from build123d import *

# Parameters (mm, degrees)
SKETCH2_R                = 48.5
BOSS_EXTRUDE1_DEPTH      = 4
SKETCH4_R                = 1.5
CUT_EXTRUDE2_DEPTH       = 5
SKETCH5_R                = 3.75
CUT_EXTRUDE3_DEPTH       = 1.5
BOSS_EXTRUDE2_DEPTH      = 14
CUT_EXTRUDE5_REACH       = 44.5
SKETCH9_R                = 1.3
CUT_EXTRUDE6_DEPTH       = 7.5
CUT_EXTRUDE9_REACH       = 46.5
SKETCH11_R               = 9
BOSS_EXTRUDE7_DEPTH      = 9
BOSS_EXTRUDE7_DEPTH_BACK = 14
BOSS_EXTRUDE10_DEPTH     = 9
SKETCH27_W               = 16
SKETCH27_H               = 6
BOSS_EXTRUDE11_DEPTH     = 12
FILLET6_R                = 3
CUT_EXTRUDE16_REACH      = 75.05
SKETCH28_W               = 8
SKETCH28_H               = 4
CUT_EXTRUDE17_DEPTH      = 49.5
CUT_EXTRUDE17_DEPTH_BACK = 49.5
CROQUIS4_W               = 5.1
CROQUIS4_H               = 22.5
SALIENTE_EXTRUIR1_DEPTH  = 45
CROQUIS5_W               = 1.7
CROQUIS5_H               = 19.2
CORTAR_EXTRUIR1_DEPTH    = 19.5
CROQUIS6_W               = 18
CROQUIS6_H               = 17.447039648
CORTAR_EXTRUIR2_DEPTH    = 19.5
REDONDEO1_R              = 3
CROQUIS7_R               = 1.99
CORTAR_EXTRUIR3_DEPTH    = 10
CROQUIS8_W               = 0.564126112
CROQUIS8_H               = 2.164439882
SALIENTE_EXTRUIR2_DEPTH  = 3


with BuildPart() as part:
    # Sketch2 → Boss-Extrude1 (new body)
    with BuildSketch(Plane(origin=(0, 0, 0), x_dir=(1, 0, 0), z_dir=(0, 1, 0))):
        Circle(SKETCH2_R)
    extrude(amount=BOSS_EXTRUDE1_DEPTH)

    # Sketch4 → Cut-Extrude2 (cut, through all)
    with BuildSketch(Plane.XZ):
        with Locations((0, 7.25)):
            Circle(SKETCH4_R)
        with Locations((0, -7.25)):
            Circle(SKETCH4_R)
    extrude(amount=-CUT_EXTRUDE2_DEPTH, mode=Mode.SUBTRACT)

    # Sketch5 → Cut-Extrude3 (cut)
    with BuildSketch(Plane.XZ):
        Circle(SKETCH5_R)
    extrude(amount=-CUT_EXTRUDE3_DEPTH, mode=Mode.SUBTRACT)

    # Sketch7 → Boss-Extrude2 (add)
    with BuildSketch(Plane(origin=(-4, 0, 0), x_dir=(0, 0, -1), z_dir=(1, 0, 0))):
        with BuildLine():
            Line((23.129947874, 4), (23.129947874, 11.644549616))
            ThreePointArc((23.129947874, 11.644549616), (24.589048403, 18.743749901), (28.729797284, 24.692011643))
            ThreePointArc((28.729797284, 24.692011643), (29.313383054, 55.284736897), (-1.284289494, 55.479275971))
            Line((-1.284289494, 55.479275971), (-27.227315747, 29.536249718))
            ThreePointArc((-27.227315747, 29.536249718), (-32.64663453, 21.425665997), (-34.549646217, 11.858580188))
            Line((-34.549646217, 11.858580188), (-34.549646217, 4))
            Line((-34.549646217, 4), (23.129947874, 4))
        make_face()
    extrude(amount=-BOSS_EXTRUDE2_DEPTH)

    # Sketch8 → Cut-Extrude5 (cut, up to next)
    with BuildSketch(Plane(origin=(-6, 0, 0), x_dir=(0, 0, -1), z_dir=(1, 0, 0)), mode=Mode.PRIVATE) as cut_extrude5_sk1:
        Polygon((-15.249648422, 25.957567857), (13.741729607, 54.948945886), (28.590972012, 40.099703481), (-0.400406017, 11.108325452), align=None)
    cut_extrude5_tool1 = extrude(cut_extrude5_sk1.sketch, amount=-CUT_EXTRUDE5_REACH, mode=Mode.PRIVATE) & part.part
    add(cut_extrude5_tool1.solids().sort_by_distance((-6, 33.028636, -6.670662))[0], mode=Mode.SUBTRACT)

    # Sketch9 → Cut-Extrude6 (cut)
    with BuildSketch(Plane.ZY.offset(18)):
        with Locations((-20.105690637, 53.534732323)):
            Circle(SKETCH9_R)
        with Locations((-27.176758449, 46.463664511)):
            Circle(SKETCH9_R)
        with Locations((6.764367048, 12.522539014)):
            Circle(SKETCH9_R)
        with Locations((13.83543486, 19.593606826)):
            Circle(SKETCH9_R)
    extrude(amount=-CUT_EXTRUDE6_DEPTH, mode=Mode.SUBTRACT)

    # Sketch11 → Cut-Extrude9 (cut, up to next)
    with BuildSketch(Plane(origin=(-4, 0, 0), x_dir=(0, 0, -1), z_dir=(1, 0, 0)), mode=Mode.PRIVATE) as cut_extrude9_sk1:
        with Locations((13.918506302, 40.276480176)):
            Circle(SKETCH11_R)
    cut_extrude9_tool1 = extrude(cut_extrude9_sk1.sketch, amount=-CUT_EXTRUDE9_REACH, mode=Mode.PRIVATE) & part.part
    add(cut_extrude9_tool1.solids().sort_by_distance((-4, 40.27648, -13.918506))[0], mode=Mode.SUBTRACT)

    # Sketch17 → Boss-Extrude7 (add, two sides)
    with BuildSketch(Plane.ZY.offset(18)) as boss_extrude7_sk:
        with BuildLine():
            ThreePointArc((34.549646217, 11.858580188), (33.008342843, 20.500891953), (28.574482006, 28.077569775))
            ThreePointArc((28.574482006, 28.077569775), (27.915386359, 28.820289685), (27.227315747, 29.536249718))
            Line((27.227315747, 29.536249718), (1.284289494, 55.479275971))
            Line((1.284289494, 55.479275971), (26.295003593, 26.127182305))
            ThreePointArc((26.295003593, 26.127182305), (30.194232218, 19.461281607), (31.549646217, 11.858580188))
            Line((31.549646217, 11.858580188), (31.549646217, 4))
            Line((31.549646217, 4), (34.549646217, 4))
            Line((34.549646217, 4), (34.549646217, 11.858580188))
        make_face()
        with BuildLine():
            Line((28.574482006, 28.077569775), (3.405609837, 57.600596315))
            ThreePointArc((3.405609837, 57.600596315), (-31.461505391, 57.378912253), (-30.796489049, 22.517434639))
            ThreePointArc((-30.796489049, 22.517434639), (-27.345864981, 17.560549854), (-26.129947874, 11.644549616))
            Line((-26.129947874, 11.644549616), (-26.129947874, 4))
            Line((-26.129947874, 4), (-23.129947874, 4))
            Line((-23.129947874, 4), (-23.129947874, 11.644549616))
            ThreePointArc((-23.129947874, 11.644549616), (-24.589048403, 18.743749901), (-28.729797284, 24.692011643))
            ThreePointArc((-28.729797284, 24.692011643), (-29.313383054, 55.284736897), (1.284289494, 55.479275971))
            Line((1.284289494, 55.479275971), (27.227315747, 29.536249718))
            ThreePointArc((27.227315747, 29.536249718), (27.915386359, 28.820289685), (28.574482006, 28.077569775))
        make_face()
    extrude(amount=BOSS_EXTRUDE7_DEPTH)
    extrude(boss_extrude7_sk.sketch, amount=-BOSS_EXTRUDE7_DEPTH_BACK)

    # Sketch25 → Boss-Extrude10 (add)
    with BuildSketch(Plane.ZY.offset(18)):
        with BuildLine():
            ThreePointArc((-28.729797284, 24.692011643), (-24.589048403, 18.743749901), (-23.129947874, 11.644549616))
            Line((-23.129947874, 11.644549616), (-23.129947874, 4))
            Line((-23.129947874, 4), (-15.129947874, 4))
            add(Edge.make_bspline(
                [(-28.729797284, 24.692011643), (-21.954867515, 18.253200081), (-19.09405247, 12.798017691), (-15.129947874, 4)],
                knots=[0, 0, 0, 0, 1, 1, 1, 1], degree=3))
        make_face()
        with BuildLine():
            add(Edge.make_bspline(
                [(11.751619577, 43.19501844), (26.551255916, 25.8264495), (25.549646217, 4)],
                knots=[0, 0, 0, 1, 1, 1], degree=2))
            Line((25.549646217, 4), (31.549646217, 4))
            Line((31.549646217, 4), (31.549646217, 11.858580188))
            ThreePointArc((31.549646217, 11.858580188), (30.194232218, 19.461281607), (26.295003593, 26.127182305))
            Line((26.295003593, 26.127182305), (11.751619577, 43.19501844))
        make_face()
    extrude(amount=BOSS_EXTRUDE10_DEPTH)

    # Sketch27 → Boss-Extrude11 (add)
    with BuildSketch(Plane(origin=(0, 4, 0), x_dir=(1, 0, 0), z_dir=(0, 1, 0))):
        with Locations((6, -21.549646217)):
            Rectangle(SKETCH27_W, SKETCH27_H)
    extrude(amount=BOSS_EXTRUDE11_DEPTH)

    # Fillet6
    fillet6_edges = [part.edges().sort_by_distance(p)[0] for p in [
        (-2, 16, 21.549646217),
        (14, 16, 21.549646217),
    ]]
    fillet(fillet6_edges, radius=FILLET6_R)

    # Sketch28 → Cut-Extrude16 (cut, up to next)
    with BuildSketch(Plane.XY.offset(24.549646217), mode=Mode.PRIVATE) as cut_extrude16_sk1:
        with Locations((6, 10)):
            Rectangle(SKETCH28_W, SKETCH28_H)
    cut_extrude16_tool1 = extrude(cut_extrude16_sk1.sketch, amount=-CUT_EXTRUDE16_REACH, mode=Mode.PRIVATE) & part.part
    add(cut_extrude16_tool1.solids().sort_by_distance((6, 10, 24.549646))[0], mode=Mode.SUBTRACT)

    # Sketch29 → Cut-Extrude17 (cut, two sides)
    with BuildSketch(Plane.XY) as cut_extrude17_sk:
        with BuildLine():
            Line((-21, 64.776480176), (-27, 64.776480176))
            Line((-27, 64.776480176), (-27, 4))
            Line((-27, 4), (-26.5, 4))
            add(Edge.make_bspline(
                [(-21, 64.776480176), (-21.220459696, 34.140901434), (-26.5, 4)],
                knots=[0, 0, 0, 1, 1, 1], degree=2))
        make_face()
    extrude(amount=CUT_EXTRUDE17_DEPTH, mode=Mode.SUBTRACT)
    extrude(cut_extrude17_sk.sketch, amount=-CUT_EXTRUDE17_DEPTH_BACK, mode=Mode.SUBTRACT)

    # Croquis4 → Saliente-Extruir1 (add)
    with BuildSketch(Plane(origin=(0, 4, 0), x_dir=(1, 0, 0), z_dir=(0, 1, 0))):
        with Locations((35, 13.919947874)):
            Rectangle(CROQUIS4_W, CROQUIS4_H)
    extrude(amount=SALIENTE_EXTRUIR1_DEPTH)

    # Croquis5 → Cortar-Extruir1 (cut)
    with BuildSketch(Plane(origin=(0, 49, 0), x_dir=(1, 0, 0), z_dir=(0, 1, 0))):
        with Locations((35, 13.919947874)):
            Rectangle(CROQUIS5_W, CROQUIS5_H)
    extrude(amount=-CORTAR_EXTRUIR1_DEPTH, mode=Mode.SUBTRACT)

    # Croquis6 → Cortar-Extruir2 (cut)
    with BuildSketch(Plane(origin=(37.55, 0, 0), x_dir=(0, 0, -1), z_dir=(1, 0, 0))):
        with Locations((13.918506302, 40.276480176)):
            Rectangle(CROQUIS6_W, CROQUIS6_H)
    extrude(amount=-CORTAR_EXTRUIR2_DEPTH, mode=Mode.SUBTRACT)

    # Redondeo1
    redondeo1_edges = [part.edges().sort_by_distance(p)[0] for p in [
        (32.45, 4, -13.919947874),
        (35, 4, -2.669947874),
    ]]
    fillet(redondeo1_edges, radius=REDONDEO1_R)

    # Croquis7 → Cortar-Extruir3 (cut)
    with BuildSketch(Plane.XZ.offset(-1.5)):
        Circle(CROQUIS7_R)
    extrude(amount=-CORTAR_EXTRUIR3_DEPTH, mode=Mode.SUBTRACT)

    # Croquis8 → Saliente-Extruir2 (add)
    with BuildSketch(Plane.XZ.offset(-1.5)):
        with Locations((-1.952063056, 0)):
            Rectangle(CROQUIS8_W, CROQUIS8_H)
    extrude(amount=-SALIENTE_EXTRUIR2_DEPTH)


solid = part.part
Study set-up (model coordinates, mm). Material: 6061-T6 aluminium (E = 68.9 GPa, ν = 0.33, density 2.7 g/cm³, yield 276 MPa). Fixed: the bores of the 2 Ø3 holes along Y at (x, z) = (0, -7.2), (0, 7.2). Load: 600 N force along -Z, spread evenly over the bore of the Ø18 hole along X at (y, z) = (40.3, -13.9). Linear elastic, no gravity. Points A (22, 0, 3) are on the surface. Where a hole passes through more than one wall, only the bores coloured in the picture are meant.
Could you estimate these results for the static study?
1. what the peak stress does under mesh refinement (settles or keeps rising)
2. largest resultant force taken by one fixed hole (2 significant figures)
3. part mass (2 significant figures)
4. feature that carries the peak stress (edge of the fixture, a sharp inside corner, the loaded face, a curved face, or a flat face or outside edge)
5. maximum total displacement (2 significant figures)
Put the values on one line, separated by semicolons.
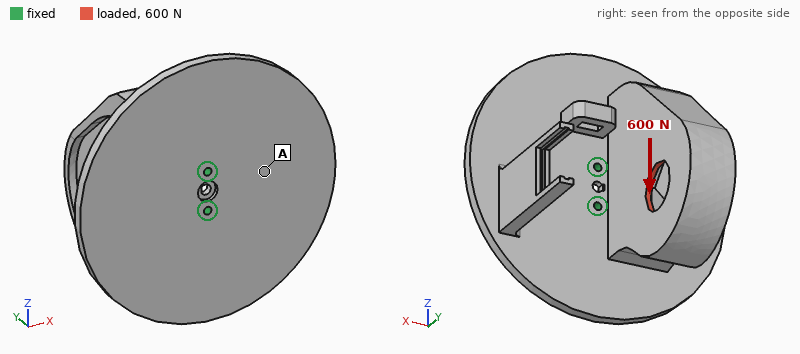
keeps rising; 1.3 kN; 190 g; edge of the fixture; 0.10 mm
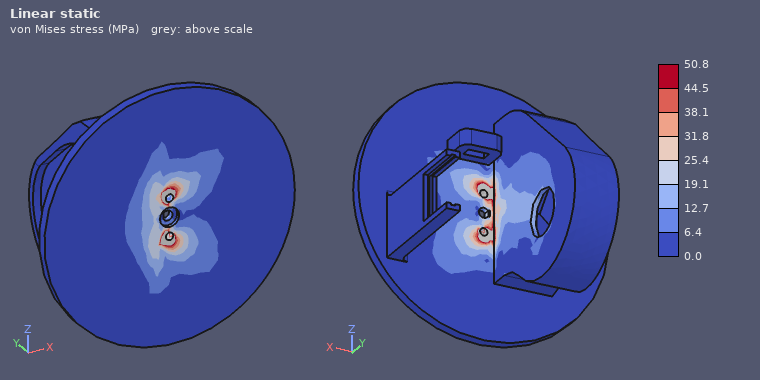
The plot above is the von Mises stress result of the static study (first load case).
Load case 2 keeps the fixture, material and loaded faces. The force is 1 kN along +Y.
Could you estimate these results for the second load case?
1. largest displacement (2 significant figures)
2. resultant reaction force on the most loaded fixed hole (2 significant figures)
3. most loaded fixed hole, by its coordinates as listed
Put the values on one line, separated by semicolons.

92 µm; 1.2 kN; (0, -7.2)
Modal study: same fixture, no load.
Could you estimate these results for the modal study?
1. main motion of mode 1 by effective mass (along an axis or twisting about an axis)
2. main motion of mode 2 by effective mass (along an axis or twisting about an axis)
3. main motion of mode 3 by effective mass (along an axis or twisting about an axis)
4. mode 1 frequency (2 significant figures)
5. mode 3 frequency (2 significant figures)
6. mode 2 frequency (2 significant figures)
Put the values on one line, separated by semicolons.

along X; along Y; along Z; 630 Hz; 1400 Hz; 1200 Hz
